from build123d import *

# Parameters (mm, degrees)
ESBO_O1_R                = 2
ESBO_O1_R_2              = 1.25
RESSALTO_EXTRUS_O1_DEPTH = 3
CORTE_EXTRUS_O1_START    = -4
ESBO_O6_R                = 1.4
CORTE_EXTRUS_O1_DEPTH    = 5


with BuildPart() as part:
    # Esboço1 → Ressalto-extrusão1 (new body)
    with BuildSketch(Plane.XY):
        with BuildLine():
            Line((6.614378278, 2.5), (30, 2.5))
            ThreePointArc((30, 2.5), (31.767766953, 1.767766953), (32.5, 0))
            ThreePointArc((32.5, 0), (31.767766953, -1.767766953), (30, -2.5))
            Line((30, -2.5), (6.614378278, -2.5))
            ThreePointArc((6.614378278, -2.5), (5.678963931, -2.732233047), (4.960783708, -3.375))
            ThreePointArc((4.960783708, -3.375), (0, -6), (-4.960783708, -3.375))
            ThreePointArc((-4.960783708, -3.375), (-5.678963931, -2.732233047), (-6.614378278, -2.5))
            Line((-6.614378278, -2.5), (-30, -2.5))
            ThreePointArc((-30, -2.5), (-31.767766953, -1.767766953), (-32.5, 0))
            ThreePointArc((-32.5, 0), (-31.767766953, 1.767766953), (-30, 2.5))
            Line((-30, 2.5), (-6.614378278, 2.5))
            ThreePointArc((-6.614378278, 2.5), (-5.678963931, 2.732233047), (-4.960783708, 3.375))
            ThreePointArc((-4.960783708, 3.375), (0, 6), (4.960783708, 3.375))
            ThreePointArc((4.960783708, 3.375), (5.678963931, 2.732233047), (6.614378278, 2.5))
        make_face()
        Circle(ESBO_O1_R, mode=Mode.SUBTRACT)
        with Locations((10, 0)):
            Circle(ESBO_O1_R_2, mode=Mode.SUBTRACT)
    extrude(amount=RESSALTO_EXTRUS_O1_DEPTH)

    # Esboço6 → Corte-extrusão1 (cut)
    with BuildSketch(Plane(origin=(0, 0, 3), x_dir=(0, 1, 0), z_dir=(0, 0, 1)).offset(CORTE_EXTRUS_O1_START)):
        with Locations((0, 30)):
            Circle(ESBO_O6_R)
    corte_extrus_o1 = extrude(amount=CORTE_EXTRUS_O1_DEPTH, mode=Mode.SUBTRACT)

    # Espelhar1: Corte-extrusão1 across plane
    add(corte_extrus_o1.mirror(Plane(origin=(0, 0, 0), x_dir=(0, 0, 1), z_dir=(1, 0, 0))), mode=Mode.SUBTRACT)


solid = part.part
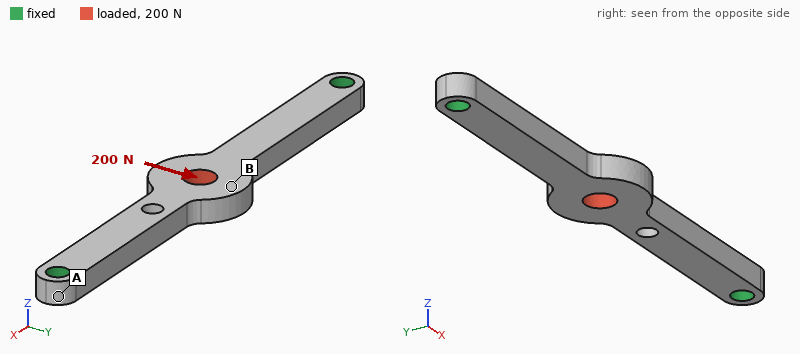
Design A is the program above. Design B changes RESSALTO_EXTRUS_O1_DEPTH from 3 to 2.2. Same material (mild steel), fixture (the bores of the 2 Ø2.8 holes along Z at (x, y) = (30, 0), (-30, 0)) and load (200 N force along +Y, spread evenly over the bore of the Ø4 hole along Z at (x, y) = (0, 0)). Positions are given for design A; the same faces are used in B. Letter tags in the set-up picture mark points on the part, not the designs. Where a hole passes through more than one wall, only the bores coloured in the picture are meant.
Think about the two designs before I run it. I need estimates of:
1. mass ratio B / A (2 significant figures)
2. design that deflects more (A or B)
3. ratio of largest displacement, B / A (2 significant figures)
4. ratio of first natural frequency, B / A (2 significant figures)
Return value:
0.73
B
1.4
0.75
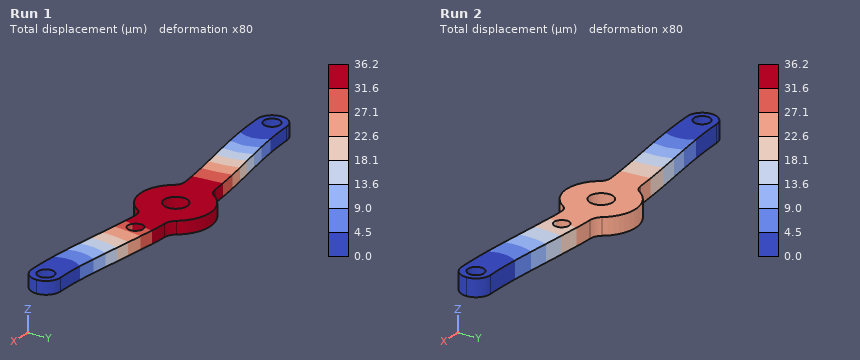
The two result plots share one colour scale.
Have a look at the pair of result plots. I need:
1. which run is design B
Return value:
Run 1
